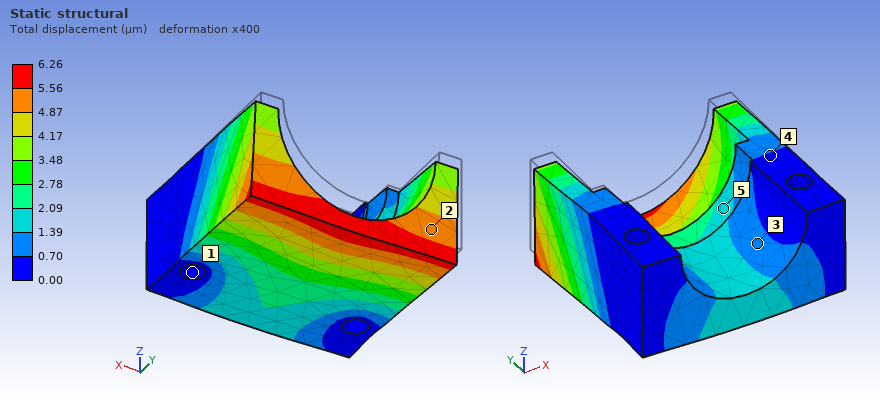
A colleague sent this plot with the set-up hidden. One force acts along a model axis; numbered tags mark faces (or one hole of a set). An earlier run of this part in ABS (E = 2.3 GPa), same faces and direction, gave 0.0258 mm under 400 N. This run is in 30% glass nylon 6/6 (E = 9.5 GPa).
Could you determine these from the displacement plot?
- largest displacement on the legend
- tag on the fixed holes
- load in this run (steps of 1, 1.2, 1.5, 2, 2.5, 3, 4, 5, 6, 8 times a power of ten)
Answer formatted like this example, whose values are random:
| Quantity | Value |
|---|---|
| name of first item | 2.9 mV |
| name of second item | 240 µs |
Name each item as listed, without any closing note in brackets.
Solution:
| Quantity | Value |
|---|---|
| largest displacement on the legend | 6.26 µm |
| tag on the fixed holes | 1 |
| load in this run | 400 N |
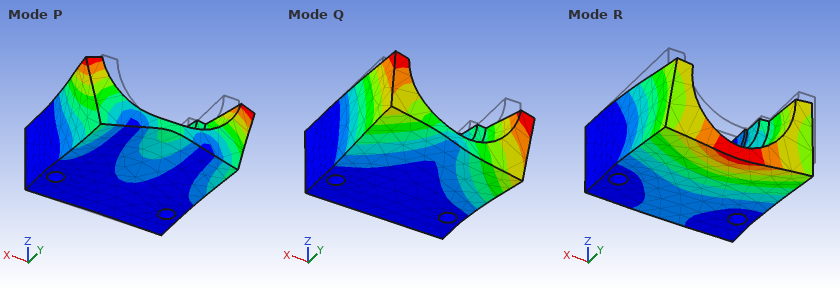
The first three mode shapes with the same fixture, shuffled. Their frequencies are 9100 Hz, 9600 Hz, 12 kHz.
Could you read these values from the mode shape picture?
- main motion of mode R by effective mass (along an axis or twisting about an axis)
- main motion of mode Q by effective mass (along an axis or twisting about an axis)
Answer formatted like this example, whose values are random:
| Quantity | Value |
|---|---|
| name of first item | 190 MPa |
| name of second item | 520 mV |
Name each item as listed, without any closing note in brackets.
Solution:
| Quantity | Value |
|---|---|
| main motion of mode R by effective mass | along Z |
| main motion of mode Q by effective mass | along X |
